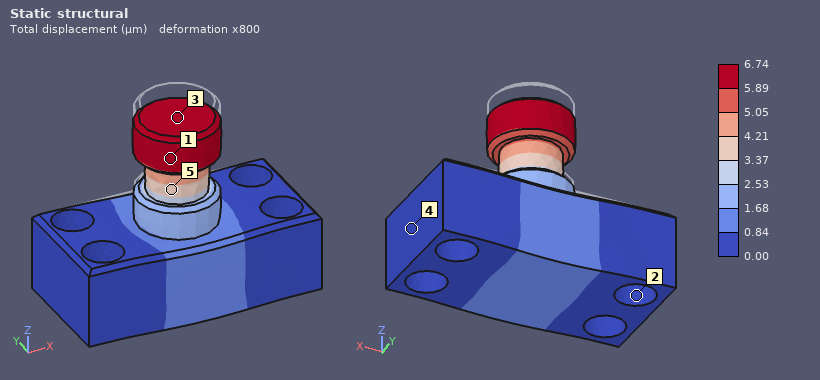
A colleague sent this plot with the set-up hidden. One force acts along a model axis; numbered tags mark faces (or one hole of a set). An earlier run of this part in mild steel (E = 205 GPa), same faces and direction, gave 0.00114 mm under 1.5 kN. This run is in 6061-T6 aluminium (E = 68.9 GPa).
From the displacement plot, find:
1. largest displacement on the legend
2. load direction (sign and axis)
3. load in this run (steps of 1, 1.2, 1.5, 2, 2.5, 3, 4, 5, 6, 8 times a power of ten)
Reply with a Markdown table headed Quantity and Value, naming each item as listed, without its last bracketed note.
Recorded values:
| Quantity | Value |
|---|---|
| largest displacement on the legend | 6.74 µm |
| load direction | -Z |
| load in this run | 3 kN |
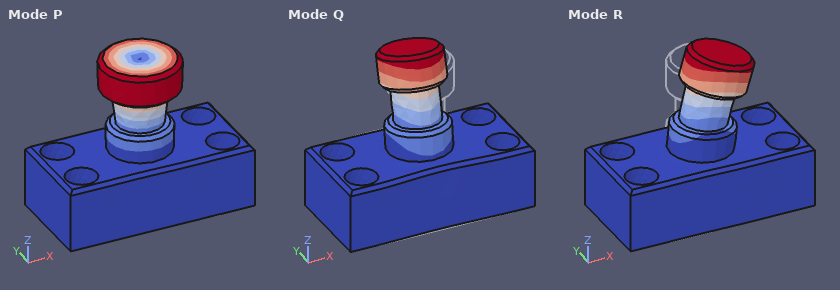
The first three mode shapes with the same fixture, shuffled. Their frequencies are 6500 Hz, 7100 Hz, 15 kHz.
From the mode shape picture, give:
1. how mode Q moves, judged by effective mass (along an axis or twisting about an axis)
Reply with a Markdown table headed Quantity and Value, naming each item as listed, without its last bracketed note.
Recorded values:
| Quantity | Value |
|---|---|
| how mode Q moves, judged by effective mass | along Y |
